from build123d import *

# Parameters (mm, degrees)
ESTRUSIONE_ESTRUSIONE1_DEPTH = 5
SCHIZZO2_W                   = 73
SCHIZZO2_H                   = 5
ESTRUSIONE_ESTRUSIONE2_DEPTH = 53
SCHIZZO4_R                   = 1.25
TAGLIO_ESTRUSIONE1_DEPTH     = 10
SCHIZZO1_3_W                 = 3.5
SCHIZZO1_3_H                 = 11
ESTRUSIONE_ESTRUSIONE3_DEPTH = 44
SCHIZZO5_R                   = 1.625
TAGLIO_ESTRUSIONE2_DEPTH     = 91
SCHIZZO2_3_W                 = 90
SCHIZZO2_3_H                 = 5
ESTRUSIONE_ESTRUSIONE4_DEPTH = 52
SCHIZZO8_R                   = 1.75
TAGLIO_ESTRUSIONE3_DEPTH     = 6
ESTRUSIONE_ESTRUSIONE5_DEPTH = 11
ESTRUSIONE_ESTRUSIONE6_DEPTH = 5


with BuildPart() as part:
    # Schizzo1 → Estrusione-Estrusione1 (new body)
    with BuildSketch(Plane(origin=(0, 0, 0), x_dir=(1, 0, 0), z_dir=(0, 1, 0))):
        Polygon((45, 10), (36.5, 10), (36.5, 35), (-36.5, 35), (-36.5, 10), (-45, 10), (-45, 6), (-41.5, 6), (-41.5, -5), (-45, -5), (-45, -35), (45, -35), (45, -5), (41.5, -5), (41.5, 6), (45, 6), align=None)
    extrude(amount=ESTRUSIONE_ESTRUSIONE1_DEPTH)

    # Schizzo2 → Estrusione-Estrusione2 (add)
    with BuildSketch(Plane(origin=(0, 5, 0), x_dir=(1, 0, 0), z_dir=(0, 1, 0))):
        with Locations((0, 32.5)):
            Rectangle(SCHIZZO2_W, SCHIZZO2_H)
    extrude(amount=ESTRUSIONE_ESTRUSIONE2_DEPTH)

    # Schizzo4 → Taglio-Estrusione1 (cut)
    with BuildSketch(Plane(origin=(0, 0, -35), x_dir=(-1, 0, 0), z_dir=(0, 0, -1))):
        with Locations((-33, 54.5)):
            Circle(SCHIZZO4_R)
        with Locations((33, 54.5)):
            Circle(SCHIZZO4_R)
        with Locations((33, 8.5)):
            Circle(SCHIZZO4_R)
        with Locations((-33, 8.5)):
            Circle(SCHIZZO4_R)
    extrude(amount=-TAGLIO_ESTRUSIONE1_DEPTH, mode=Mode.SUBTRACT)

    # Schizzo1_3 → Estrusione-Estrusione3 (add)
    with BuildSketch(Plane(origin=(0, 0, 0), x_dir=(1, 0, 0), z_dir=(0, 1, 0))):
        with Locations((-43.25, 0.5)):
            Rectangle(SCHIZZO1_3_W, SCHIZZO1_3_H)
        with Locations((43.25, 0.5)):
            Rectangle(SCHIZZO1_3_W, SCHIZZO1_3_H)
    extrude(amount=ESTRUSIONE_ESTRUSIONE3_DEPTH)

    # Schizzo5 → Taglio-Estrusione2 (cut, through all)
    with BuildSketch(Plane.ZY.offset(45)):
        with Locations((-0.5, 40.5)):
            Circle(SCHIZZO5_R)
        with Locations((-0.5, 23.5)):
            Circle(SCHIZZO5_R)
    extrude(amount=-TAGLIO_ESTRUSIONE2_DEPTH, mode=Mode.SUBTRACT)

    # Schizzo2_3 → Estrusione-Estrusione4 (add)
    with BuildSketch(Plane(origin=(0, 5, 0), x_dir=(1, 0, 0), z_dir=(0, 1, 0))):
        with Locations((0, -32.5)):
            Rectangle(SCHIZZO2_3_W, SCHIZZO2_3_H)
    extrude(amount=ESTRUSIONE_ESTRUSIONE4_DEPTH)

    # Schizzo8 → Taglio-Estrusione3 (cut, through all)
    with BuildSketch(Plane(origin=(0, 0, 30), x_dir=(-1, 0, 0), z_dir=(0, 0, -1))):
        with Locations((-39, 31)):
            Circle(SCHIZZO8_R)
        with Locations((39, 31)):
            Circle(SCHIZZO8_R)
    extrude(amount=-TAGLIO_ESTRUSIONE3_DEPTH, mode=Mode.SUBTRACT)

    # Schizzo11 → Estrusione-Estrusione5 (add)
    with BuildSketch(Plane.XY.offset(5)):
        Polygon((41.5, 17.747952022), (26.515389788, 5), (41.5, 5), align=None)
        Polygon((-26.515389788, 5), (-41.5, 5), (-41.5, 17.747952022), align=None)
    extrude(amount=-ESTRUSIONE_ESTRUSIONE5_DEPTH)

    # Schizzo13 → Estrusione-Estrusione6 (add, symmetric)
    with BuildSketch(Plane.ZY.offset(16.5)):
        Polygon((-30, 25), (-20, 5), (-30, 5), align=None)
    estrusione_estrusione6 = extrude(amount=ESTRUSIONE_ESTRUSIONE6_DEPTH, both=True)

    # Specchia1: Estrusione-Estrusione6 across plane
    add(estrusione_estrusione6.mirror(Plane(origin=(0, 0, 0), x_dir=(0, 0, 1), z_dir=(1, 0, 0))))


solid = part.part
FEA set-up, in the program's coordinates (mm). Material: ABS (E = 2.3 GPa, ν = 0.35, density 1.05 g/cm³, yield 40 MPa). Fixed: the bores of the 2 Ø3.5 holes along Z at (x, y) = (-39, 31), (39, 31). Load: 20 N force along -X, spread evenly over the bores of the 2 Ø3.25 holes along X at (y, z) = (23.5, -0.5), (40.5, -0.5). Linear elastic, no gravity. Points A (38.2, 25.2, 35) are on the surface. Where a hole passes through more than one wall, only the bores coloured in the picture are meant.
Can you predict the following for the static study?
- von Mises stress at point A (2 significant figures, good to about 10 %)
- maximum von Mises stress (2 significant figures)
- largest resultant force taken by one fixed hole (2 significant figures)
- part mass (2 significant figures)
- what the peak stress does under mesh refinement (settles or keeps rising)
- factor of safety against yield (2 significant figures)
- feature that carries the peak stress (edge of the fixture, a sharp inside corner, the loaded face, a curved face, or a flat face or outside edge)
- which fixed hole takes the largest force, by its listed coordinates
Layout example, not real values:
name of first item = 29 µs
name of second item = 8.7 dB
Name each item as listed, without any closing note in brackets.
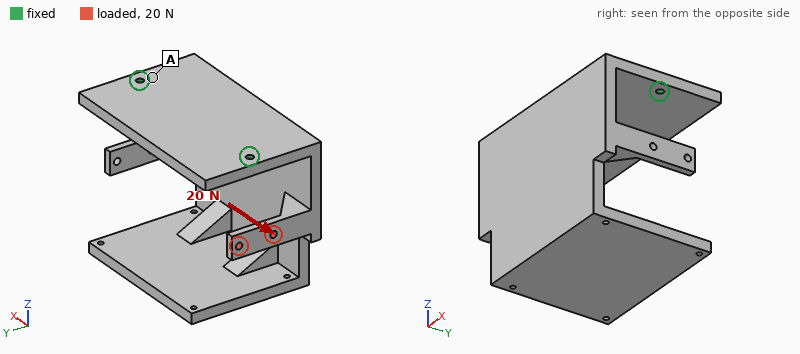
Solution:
von Mises stress at point A = 1.6 MPa
maximum von Mises stress = 18 MPa
largest resultant force taken by one fixed hole = 15 N
part mass = 83 g
what the peak stress does under mesh refinement = settles
factor of safety against yield = 2.2
feature that carries the peak stress = the loaded face
which fixed hole takes the largest force, by its listed coordinates = (-39, 31)
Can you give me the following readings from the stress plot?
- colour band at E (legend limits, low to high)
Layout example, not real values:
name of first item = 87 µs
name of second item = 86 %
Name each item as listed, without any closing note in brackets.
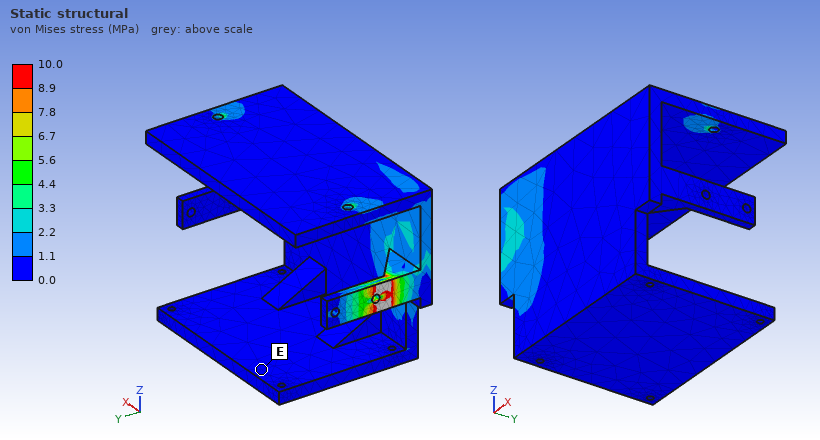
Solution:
colour band at E = 0.0 to 1.1 MPa
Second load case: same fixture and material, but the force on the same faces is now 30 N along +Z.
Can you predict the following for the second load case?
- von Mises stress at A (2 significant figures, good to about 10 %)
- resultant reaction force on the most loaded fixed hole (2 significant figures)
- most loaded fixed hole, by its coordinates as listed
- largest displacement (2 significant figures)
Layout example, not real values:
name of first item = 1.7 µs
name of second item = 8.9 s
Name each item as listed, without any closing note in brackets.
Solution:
von Mises stress at A = 2.4 MPa
resultant reaction force on the most loaded fixed hole = 33 N
most loaded fixed hole, by its coordinates as listed = (-39, 31)
largest displacement = 1.5 mm
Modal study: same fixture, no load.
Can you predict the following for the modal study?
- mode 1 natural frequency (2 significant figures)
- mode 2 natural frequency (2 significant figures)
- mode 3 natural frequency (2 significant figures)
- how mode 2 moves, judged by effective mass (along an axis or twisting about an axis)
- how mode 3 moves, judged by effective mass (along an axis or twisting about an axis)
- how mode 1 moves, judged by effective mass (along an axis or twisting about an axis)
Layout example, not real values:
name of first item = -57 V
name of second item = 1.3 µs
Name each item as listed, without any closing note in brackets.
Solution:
mode 1 natural frequency = 81 Hz
mode 2 natural frequency = 170 Hz
mode 3 natural frequency = 250 Hz
how mode 2 moves, judged by effective mass = along X
how mode 3 moves, judged by effective mass = along Z
how mode 1 moves, judged by effective mass = along Y
